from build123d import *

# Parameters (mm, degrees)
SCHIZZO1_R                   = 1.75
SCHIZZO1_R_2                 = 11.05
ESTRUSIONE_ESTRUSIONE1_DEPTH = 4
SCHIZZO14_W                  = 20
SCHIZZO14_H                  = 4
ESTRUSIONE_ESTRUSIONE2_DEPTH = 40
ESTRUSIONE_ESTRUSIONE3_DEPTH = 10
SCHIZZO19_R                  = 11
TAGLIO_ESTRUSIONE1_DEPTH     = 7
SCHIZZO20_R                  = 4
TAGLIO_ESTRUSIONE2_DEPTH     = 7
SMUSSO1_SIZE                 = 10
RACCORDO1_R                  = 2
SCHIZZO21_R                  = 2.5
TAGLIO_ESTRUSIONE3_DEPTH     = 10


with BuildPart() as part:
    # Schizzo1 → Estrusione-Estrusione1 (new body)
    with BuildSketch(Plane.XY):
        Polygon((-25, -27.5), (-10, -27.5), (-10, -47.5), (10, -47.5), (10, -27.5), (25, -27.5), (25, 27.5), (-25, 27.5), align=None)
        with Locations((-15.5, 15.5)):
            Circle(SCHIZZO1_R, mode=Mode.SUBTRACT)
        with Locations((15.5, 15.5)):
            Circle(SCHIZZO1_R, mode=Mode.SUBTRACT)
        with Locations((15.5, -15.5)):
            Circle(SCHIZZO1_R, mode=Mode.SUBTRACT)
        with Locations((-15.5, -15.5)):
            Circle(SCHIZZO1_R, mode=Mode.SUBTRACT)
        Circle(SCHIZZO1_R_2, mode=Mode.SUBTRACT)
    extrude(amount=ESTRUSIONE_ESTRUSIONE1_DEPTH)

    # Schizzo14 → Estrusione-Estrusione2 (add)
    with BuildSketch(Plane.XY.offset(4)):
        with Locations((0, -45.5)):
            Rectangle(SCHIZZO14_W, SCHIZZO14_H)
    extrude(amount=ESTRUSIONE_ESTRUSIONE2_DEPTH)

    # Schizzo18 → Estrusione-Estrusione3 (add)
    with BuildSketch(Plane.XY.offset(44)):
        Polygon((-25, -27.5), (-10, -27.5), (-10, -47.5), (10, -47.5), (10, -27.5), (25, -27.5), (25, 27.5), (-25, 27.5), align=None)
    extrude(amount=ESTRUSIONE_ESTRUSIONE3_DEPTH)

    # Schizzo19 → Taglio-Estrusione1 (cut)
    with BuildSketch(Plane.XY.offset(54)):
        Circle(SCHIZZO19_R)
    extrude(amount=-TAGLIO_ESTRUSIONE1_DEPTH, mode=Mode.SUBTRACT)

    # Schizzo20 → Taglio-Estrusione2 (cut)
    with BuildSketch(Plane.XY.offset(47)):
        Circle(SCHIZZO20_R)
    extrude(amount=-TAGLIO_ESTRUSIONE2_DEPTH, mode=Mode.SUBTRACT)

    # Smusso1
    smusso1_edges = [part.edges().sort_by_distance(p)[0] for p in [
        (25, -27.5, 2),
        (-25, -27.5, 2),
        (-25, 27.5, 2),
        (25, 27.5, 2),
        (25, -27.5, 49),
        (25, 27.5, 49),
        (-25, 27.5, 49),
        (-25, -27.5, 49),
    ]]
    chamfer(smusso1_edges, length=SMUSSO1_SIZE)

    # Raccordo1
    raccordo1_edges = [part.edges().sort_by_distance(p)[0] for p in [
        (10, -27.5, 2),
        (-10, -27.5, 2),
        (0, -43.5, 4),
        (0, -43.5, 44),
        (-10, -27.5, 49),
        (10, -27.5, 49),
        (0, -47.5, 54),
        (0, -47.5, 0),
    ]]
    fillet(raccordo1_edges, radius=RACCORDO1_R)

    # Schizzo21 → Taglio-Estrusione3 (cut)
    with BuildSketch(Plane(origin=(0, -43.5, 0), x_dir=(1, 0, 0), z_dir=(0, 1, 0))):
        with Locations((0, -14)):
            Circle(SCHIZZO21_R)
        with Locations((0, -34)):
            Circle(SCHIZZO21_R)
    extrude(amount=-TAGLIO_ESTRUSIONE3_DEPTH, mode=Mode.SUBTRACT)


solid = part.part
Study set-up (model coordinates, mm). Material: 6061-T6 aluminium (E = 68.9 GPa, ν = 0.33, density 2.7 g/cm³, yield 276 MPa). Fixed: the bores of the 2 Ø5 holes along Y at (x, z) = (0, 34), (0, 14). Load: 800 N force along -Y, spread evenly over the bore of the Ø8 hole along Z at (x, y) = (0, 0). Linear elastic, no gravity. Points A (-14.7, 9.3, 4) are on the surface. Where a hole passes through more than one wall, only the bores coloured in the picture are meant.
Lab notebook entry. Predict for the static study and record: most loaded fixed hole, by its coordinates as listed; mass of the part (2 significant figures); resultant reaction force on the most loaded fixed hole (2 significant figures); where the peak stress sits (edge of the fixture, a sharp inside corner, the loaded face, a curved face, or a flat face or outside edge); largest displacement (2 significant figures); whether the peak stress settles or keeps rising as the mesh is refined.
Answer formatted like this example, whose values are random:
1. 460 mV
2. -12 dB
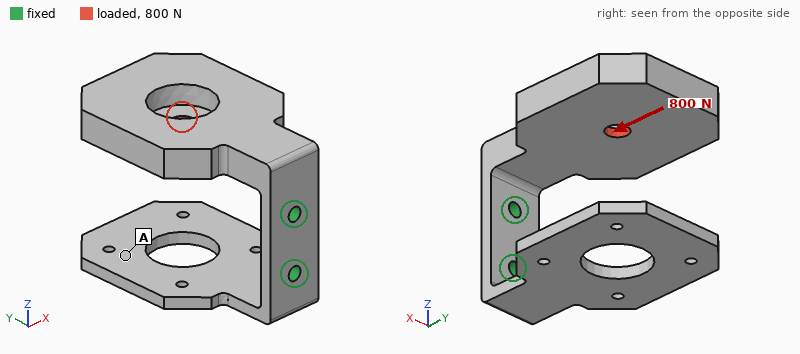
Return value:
1. (0, 34)
2. 110 g
3. 870 N
4. edge of the fixture
5. 0.42 mm
6. keeps rising
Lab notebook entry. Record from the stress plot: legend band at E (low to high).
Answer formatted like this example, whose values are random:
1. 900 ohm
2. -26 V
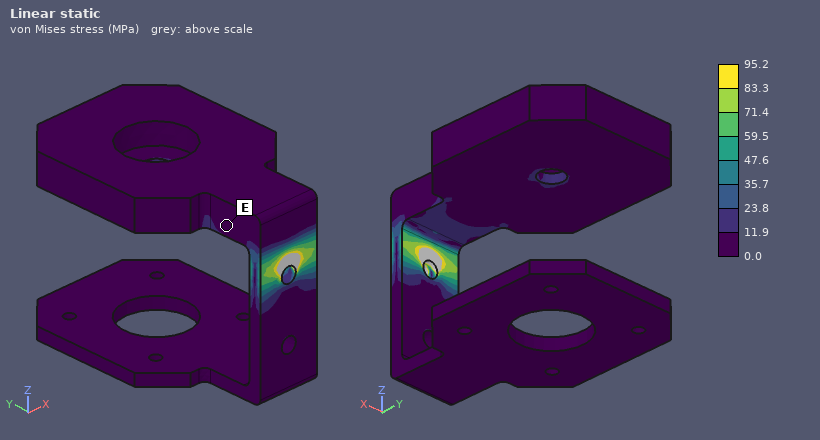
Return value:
1. 0.0 to 11.9 MPa
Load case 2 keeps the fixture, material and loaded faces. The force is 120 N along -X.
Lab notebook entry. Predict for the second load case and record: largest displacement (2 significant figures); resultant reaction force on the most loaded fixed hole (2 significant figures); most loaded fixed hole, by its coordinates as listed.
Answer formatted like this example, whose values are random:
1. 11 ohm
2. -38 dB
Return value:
1. 0.29 mm
2. 160 N
3. (0, 34)
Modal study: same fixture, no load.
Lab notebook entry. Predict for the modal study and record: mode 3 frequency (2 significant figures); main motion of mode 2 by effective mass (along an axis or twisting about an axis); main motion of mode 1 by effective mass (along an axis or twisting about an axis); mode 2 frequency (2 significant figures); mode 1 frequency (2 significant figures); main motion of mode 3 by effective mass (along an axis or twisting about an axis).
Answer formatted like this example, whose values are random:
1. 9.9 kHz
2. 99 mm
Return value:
1. 480 Hz
2. along Z
3. along Z
4. 380 Hz
5. 340 Hz
6. along X
